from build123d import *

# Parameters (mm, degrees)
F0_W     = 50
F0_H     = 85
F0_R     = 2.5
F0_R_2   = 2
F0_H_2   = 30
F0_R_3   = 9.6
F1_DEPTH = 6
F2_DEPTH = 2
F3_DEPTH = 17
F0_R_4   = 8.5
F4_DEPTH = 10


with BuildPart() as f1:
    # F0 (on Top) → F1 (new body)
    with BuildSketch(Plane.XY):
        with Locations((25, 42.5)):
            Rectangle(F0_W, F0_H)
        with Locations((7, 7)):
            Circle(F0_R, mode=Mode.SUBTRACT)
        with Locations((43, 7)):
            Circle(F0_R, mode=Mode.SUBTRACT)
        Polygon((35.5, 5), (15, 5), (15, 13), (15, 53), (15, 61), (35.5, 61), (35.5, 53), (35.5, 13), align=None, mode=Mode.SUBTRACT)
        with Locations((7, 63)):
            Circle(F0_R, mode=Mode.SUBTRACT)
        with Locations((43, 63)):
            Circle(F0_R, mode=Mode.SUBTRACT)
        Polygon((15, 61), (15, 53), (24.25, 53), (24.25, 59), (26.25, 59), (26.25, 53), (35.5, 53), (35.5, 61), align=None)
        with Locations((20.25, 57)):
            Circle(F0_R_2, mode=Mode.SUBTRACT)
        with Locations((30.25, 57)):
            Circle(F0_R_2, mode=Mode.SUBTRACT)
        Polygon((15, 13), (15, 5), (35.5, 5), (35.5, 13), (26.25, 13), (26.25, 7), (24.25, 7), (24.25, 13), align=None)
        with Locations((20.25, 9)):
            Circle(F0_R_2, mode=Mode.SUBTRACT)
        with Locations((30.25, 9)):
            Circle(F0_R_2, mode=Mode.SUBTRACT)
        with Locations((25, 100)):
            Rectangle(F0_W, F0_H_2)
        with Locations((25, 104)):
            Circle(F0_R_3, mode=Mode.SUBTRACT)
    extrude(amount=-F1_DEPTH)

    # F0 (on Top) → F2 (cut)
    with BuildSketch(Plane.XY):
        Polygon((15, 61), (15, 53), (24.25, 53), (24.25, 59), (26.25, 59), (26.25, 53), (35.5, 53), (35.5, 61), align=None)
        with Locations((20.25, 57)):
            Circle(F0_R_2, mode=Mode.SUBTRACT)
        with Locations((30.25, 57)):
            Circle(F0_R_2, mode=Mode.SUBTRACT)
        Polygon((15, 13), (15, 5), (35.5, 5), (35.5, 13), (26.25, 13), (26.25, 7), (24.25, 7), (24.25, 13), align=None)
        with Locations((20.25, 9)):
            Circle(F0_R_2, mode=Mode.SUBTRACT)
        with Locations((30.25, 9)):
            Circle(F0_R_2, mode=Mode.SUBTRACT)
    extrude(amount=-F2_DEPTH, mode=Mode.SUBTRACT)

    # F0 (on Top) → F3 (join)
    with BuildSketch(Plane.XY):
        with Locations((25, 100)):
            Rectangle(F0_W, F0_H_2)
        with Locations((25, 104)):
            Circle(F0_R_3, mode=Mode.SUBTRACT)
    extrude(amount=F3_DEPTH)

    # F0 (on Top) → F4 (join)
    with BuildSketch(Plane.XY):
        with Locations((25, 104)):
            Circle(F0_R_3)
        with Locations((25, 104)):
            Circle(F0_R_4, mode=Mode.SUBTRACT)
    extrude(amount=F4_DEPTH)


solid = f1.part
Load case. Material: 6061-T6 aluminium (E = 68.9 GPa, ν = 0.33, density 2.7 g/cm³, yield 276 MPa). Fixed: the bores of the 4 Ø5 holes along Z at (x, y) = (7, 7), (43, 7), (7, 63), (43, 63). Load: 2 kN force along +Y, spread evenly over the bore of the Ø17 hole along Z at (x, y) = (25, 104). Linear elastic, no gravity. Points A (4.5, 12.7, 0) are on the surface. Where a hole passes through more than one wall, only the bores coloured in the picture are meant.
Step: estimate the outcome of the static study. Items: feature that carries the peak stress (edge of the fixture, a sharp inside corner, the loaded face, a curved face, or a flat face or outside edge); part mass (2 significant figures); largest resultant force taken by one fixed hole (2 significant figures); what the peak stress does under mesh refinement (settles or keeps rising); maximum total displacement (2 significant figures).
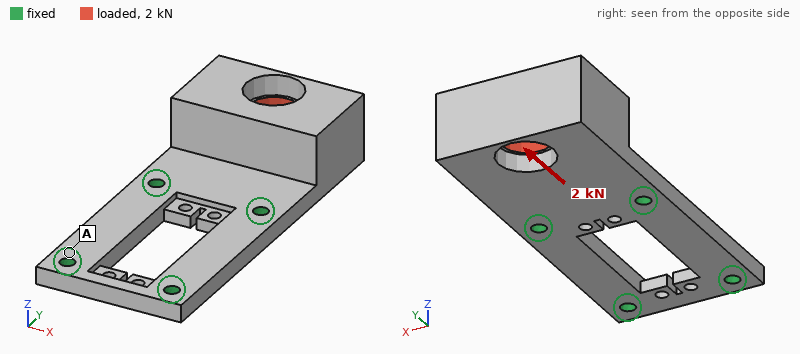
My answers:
edge of the fixture
130 g
990 N
keeps rising
0.29 mm
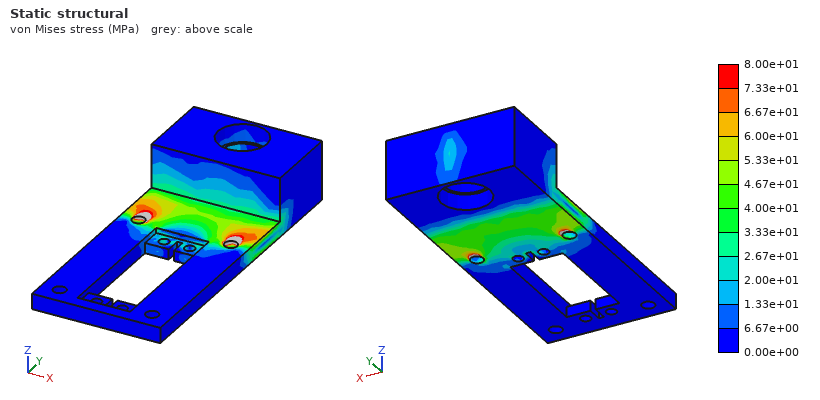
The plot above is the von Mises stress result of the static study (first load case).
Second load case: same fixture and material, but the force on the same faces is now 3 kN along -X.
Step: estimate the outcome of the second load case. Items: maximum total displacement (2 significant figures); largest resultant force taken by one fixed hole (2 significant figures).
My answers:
86 µm
3.5 kN
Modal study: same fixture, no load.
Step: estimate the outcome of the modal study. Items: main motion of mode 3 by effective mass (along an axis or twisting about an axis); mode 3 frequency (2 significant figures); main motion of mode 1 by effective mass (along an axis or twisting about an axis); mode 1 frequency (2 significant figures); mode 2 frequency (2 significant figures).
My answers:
along X
5800 Hz
along Z
980 Hz
3100 Hz
